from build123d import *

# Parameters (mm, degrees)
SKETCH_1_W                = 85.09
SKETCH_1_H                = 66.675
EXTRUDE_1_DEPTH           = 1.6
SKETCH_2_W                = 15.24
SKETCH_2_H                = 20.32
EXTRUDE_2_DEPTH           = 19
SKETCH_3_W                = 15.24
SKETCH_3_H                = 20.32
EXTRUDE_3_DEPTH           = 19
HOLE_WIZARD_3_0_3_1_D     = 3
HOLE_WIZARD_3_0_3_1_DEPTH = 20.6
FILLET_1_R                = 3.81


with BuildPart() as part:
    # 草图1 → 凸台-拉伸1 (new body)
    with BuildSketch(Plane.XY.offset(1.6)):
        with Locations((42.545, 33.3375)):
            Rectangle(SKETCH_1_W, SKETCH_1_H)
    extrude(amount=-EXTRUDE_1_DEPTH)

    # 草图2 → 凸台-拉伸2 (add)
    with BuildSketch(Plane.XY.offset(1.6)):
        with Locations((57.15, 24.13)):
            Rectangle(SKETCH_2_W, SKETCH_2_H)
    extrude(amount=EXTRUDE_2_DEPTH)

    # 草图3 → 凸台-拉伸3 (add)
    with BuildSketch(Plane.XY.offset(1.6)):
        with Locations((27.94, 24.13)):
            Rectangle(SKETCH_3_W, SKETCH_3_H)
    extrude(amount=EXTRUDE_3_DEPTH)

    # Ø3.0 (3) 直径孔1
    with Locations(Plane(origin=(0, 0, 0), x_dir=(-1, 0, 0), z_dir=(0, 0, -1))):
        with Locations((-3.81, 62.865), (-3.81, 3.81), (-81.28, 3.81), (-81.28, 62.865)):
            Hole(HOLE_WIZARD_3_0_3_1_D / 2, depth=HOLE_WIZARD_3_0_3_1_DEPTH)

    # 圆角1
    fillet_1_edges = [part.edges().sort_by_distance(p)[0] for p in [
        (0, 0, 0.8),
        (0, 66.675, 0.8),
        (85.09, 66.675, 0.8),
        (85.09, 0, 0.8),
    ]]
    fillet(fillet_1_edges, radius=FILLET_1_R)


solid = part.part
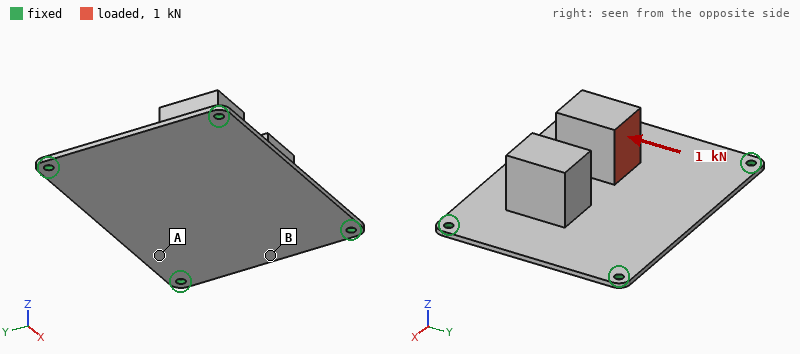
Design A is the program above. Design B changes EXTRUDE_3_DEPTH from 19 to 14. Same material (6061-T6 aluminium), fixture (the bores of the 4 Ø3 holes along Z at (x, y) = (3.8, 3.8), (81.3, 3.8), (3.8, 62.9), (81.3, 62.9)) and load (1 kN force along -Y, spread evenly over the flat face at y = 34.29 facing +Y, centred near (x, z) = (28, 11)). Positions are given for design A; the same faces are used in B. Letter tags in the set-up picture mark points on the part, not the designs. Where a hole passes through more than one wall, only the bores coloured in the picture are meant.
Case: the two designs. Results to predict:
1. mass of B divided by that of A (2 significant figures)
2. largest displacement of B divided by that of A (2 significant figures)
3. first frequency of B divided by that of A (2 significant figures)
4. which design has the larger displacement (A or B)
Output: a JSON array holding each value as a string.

["0.93", "0.64", "1.1", "A"]
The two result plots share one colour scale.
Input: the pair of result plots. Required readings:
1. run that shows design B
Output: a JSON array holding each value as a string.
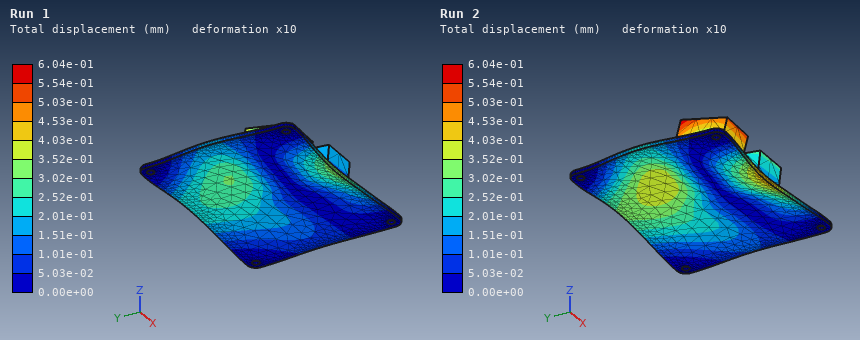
["Run 1"]
